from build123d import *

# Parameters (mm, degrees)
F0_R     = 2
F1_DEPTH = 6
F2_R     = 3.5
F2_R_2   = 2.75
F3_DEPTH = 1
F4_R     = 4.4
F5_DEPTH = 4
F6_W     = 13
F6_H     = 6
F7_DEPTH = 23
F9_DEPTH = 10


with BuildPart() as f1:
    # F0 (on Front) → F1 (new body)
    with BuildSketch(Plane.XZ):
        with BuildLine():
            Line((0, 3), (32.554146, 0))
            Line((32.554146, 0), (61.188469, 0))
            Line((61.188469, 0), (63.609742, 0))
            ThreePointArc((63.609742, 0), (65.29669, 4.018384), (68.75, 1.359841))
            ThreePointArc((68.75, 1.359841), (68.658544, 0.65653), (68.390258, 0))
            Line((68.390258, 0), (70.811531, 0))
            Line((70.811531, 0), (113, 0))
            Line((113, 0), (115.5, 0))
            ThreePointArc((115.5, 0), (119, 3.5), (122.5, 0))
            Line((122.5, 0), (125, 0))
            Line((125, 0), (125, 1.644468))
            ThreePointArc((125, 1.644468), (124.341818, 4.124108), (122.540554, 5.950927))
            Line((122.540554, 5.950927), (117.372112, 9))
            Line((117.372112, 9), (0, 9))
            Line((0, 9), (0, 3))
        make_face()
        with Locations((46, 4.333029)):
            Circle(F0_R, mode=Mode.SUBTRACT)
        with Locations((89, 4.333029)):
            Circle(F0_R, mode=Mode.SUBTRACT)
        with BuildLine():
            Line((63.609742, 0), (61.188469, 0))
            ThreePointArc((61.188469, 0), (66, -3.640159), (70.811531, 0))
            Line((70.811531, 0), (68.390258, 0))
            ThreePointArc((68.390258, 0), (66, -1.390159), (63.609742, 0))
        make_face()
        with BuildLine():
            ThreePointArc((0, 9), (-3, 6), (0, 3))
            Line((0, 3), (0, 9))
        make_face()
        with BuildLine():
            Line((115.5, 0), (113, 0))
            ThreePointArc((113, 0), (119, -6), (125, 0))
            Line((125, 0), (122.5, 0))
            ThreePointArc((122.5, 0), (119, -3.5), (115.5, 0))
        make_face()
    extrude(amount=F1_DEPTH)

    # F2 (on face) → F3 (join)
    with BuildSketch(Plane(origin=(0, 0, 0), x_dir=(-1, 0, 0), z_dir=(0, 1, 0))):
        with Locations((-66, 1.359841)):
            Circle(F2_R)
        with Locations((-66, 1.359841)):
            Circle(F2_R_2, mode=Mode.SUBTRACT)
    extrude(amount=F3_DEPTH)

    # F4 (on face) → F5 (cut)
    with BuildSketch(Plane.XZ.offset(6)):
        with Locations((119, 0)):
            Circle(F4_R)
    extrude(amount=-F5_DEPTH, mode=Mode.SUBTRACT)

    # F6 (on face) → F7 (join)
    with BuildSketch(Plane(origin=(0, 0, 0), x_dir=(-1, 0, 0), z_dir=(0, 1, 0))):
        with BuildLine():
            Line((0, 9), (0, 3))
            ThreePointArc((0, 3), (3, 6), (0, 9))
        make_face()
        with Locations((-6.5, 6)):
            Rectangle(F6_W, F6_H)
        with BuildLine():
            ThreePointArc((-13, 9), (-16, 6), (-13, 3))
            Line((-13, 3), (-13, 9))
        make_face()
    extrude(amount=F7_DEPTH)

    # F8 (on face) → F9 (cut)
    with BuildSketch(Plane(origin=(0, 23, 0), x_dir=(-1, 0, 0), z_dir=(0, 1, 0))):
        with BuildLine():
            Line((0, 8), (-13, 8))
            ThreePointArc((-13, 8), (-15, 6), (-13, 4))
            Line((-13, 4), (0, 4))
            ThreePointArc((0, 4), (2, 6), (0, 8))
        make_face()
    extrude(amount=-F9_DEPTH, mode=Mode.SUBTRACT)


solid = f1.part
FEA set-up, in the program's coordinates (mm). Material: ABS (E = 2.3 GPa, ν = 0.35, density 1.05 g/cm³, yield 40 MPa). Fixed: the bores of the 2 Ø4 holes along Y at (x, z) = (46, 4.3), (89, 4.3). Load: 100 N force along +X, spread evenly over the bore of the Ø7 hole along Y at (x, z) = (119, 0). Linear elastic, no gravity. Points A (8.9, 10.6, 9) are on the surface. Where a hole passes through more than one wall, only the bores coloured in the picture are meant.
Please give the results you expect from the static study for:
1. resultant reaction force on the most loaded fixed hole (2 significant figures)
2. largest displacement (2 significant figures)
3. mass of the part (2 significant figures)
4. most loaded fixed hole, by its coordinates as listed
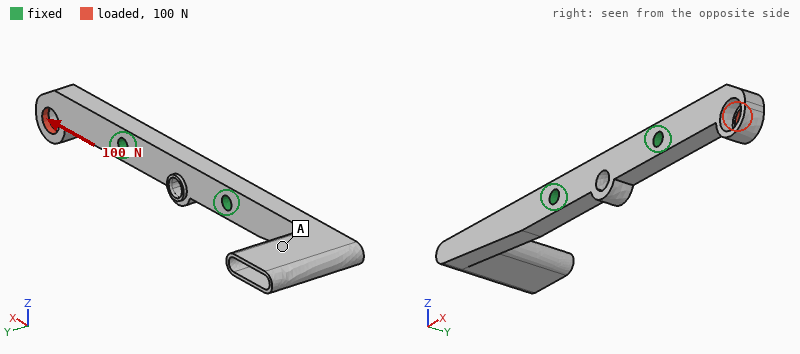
100 N
0.57 mm
8.5 g
(89, 4.3)
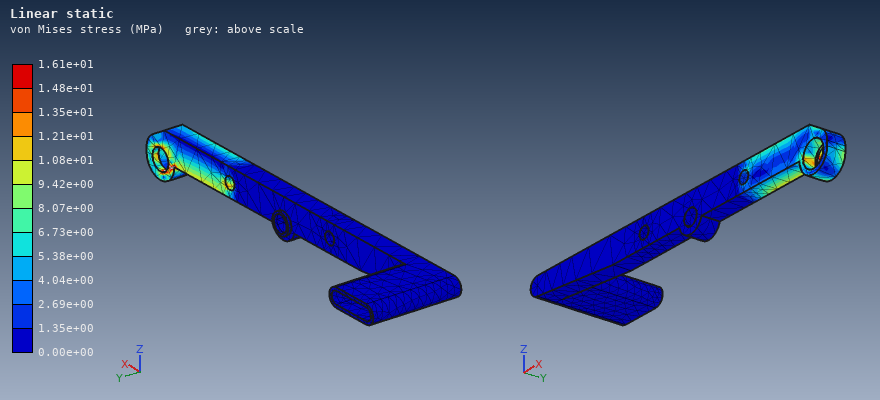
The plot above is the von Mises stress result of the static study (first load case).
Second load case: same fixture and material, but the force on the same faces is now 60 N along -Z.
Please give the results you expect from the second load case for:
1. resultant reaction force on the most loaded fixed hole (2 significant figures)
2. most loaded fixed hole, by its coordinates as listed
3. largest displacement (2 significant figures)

68 N
(89, 4.3)
1.1 mm
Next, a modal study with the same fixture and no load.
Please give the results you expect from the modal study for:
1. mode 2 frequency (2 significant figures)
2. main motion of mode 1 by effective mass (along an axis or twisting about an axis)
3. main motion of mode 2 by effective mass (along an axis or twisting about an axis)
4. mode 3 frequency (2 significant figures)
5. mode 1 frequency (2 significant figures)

480 Hz
along Y
along Z
1200 Hz
370 Hz
